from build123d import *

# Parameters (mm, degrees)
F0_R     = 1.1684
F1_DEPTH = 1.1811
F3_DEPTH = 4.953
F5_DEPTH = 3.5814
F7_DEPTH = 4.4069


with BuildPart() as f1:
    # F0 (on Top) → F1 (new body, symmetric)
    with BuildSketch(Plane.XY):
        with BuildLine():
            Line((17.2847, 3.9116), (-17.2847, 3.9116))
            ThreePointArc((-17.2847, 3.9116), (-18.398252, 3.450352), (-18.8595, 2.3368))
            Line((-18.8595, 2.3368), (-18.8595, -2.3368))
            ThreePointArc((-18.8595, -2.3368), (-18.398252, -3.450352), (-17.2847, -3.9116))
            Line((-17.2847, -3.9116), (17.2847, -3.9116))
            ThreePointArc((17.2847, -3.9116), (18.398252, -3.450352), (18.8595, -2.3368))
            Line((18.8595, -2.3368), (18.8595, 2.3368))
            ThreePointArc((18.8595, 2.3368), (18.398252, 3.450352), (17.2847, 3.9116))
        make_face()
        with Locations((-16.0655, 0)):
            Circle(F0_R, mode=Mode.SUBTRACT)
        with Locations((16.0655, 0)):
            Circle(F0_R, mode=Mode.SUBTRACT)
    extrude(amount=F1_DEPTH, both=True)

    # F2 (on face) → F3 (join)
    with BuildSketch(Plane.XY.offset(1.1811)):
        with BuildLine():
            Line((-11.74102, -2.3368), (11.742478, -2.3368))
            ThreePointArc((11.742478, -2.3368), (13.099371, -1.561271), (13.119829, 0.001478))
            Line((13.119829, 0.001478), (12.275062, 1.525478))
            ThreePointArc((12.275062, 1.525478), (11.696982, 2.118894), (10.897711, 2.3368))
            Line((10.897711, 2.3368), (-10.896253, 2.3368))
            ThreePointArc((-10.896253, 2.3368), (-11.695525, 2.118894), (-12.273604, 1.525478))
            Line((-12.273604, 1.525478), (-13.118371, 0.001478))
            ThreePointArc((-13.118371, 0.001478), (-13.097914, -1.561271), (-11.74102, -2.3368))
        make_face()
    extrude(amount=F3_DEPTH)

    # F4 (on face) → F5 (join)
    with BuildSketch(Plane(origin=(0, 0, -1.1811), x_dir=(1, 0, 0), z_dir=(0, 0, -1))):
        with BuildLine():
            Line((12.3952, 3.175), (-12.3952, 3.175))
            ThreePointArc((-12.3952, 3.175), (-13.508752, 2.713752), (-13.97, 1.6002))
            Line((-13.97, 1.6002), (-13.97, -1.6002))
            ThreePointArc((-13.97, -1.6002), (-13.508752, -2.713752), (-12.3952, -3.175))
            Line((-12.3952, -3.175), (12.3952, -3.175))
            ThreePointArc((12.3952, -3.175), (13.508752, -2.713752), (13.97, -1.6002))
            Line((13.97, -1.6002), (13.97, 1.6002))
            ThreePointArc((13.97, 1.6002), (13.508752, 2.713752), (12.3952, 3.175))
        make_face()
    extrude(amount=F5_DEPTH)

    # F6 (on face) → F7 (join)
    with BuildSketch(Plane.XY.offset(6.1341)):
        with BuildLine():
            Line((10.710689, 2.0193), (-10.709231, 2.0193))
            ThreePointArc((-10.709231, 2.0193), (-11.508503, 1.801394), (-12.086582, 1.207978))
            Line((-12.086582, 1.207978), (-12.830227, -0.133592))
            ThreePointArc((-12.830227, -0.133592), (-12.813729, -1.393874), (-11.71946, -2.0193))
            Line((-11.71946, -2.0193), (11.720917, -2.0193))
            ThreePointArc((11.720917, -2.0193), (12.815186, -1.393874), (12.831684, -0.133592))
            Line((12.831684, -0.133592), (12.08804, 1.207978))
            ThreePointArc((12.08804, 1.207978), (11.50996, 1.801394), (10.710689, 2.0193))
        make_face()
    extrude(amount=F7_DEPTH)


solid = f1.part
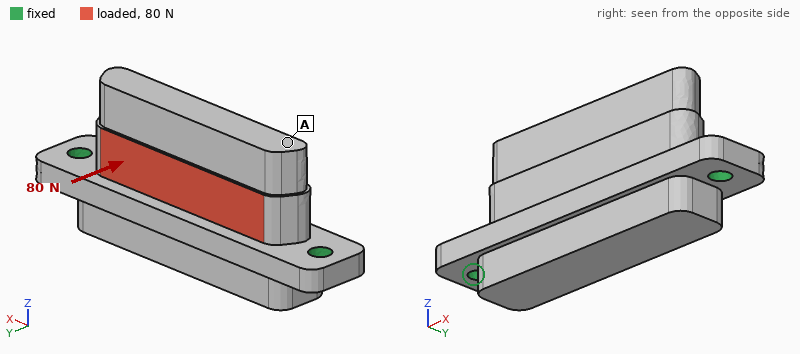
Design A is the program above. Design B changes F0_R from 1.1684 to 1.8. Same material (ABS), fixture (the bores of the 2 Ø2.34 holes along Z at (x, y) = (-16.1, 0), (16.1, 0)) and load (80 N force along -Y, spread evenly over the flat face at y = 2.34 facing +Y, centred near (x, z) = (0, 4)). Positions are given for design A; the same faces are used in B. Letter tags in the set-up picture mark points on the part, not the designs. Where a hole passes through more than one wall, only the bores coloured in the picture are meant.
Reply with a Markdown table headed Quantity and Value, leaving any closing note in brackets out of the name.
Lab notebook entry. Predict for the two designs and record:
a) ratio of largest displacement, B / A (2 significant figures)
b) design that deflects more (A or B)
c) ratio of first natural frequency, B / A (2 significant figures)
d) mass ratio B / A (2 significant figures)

| Quantity | Value |
|---|---|
| ratio of largest displacement, B / A | 0.73 |
| design that deflects more | A |
| ratio of first natural frequency, B / A | 1.2 |
| mass ratio B / A | 0.99 |
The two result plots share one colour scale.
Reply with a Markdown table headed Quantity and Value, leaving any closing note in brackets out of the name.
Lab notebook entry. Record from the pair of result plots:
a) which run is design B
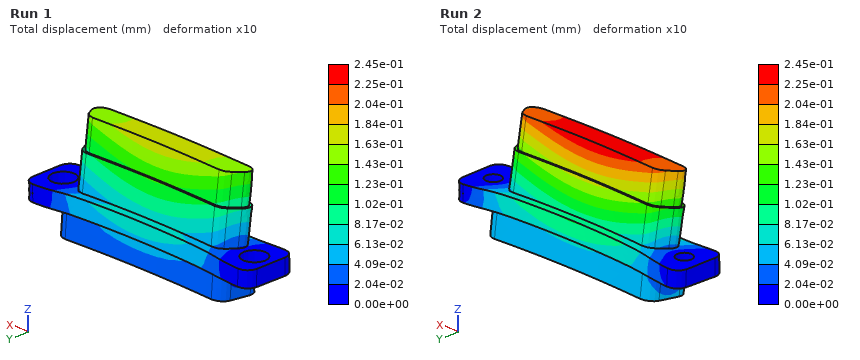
| Quantity | Value |
|---|---|
| which run is design B | Run 1 |
